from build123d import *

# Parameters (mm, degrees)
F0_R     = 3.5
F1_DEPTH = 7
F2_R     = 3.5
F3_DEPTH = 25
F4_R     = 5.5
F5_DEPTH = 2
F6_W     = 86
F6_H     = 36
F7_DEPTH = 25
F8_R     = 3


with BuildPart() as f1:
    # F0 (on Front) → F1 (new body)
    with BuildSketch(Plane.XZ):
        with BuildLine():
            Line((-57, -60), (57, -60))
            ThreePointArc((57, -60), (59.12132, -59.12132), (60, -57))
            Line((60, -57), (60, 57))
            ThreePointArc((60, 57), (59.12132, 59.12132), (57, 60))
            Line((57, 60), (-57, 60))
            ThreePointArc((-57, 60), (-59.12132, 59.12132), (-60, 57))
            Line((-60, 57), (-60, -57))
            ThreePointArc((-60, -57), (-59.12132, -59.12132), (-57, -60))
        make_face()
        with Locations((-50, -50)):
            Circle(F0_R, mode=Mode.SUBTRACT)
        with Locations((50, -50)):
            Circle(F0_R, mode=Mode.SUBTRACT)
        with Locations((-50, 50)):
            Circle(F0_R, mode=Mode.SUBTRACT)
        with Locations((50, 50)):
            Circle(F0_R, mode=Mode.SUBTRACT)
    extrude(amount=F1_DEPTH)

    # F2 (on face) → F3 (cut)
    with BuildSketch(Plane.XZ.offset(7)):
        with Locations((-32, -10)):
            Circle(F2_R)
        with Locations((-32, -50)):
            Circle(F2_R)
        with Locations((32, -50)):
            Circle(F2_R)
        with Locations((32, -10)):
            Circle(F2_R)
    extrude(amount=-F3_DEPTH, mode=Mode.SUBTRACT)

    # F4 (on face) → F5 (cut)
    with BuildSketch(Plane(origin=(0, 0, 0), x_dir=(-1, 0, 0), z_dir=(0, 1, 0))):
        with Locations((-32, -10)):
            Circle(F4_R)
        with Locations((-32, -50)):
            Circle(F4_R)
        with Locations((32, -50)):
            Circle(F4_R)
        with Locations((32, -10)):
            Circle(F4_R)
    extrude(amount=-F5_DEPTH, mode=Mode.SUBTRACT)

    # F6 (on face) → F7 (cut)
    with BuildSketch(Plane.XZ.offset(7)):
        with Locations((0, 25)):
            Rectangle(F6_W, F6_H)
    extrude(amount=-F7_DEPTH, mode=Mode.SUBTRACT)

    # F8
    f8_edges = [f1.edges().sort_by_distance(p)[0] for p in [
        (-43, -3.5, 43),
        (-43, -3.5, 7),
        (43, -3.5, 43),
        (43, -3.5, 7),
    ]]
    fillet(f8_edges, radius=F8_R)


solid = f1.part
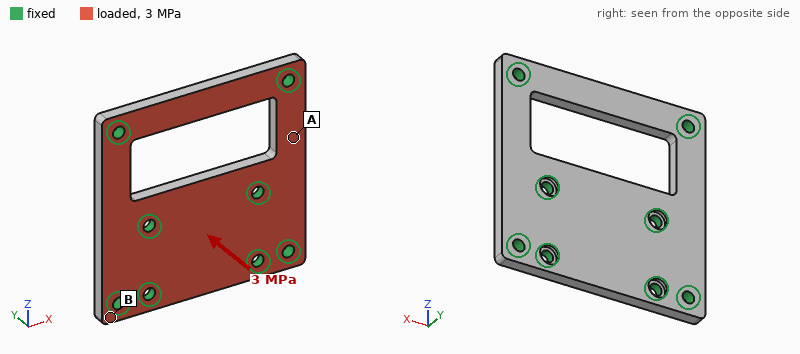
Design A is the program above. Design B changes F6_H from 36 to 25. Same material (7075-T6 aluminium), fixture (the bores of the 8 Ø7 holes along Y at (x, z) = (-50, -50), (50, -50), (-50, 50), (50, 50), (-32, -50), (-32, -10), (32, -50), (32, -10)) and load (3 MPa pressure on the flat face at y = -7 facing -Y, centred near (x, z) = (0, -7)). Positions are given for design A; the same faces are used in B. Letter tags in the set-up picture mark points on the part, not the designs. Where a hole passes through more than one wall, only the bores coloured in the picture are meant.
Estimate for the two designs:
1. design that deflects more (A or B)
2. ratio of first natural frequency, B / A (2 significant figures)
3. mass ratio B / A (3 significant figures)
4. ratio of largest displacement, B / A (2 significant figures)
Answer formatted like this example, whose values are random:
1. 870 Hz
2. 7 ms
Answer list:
1. B
2. 0.97
3. 1.09
4. 1.1
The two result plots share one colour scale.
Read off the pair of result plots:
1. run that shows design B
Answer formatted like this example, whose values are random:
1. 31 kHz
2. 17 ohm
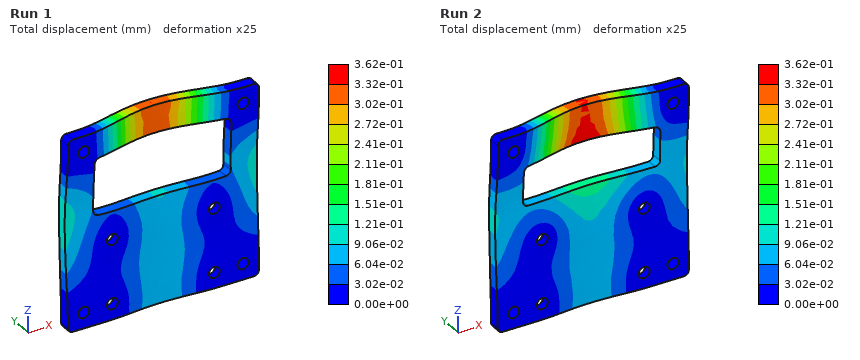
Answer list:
1. Run 2
